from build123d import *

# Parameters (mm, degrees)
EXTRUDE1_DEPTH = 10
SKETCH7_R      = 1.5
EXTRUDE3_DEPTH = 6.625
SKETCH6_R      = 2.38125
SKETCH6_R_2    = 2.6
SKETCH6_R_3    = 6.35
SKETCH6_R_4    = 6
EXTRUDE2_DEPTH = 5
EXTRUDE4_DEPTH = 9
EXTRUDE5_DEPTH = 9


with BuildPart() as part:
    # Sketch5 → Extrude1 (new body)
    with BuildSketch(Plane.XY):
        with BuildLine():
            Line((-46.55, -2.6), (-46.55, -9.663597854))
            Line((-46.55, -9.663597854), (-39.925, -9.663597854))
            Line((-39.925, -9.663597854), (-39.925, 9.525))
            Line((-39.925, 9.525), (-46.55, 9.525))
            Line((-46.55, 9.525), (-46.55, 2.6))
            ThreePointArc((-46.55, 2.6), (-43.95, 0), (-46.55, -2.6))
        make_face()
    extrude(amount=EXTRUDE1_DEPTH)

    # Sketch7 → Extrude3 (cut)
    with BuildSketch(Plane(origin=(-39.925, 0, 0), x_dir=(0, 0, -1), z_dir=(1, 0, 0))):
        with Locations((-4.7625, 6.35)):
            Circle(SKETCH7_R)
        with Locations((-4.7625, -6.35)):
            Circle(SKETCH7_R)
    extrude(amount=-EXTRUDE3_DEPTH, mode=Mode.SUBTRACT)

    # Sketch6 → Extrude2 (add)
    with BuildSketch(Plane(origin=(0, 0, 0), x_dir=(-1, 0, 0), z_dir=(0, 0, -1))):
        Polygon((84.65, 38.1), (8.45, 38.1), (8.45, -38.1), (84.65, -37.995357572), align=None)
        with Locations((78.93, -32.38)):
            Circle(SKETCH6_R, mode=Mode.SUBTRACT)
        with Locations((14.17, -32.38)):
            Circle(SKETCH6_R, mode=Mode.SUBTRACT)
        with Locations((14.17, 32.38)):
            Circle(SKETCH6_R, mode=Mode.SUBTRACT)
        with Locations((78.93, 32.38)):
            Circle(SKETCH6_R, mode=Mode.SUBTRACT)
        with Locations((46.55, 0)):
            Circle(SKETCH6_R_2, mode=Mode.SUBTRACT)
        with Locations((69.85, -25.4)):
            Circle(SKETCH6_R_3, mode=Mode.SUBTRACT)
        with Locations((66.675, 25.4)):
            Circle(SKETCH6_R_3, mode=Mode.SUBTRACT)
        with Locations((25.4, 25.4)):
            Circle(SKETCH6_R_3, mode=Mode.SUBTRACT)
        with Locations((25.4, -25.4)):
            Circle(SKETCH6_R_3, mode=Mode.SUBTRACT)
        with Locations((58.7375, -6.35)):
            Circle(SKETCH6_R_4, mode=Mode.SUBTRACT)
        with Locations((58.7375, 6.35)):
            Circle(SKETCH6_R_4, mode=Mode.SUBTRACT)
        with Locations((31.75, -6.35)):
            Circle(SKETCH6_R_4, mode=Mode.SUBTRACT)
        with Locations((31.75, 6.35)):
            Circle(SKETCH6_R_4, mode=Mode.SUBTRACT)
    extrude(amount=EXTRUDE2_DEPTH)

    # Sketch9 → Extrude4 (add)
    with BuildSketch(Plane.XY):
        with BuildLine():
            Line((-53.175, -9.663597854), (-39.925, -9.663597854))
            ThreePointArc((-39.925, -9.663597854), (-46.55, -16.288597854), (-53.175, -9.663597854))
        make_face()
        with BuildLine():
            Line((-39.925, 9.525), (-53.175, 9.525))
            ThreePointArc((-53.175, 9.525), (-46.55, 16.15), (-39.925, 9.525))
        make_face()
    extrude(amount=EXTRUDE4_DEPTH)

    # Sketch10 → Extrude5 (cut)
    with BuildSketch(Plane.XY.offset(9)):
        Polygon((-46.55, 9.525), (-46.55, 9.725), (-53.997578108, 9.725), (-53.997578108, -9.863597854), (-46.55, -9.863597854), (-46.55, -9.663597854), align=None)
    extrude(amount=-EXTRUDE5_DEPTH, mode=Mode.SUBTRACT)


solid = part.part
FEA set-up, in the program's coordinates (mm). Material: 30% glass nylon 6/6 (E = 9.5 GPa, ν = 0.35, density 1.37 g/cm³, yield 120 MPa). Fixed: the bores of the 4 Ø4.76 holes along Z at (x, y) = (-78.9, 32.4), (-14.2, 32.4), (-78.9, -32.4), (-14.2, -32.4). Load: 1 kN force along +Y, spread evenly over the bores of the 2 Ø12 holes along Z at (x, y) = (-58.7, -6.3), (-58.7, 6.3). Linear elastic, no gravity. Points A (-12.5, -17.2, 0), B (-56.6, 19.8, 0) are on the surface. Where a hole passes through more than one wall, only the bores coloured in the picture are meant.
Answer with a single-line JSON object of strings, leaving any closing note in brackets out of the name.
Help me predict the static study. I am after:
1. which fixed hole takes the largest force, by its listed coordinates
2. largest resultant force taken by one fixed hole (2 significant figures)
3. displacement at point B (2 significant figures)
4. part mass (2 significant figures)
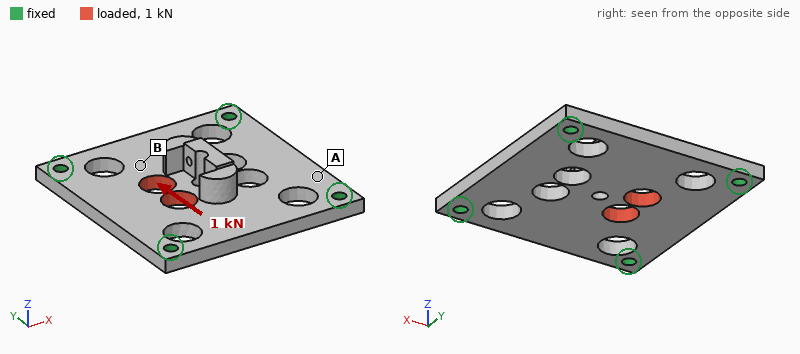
{"which fixed hole takes the largest force, by its listed coordinates": "(-78.9, 32.4)", "largest resultant force taken by one fixed hole": "390 N", "displacement at point B": "24 µm", "part mass": "36 g"}
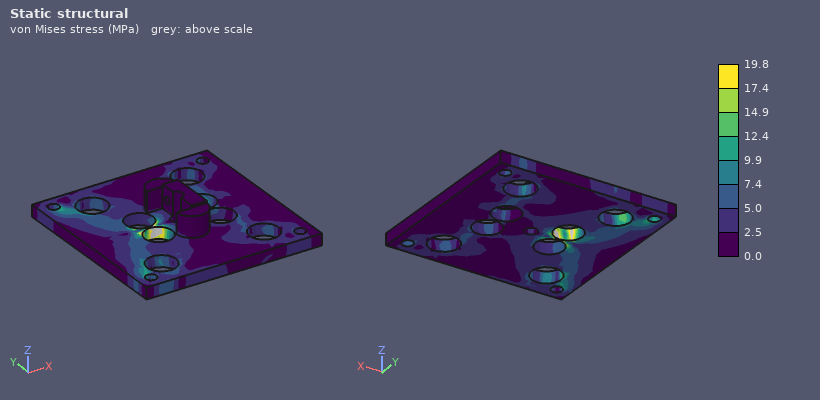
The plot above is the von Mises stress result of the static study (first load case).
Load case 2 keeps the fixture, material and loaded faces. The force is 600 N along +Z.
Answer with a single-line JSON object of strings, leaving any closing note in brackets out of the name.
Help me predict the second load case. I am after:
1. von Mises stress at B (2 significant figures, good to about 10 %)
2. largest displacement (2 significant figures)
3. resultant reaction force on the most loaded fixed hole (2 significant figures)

{"von Mises stress at B": "16 MPa", "largest displacement": "0.45 mm", "resultant reaction force on the most loaded fixed hole": "230 N"}
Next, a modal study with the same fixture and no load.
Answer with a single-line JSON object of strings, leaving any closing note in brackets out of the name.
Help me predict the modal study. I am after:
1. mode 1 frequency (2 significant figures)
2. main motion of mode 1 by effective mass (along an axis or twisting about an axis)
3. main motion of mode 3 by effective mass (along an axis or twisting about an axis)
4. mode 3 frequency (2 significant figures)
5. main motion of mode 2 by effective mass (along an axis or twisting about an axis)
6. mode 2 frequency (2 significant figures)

{"mode 1 frequency": "1800 Hz", "main motion of mode 1 by effective mass": "along Z", "main motion of mode 3 by effective mass": "twisting about Y", "mode 3 frequency": "3300 Hz", "main motion of mode 2 by effective mass": "twisting about X", "mode 2 frequency": "3100 Hz"}
